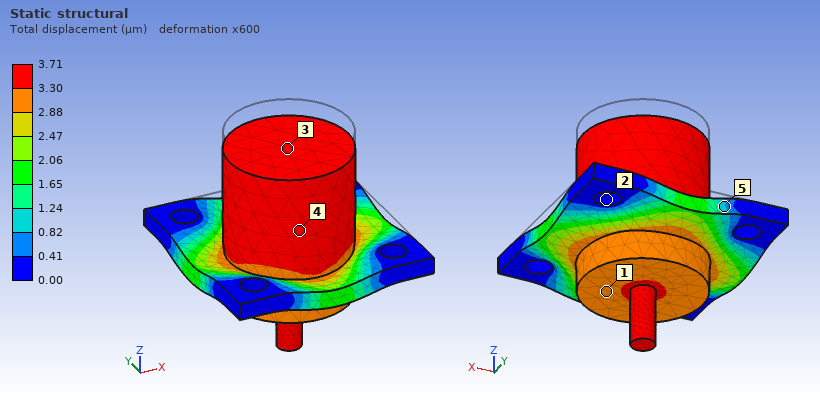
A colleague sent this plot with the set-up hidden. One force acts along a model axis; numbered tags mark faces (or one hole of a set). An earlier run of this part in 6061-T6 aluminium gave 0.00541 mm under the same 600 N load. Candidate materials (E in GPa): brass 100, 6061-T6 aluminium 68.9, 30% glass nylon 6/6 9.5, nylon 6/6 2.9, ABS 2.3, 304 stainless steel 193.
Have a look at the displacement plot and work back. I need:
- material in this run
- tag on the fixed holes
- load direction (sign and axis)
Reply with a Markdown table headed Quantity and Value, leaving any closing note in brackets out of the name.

| Quantity | Value |
|---|---|
| material in this run | brass |
| tag on the fixed holes | 2 |
| load direction | -Z |
